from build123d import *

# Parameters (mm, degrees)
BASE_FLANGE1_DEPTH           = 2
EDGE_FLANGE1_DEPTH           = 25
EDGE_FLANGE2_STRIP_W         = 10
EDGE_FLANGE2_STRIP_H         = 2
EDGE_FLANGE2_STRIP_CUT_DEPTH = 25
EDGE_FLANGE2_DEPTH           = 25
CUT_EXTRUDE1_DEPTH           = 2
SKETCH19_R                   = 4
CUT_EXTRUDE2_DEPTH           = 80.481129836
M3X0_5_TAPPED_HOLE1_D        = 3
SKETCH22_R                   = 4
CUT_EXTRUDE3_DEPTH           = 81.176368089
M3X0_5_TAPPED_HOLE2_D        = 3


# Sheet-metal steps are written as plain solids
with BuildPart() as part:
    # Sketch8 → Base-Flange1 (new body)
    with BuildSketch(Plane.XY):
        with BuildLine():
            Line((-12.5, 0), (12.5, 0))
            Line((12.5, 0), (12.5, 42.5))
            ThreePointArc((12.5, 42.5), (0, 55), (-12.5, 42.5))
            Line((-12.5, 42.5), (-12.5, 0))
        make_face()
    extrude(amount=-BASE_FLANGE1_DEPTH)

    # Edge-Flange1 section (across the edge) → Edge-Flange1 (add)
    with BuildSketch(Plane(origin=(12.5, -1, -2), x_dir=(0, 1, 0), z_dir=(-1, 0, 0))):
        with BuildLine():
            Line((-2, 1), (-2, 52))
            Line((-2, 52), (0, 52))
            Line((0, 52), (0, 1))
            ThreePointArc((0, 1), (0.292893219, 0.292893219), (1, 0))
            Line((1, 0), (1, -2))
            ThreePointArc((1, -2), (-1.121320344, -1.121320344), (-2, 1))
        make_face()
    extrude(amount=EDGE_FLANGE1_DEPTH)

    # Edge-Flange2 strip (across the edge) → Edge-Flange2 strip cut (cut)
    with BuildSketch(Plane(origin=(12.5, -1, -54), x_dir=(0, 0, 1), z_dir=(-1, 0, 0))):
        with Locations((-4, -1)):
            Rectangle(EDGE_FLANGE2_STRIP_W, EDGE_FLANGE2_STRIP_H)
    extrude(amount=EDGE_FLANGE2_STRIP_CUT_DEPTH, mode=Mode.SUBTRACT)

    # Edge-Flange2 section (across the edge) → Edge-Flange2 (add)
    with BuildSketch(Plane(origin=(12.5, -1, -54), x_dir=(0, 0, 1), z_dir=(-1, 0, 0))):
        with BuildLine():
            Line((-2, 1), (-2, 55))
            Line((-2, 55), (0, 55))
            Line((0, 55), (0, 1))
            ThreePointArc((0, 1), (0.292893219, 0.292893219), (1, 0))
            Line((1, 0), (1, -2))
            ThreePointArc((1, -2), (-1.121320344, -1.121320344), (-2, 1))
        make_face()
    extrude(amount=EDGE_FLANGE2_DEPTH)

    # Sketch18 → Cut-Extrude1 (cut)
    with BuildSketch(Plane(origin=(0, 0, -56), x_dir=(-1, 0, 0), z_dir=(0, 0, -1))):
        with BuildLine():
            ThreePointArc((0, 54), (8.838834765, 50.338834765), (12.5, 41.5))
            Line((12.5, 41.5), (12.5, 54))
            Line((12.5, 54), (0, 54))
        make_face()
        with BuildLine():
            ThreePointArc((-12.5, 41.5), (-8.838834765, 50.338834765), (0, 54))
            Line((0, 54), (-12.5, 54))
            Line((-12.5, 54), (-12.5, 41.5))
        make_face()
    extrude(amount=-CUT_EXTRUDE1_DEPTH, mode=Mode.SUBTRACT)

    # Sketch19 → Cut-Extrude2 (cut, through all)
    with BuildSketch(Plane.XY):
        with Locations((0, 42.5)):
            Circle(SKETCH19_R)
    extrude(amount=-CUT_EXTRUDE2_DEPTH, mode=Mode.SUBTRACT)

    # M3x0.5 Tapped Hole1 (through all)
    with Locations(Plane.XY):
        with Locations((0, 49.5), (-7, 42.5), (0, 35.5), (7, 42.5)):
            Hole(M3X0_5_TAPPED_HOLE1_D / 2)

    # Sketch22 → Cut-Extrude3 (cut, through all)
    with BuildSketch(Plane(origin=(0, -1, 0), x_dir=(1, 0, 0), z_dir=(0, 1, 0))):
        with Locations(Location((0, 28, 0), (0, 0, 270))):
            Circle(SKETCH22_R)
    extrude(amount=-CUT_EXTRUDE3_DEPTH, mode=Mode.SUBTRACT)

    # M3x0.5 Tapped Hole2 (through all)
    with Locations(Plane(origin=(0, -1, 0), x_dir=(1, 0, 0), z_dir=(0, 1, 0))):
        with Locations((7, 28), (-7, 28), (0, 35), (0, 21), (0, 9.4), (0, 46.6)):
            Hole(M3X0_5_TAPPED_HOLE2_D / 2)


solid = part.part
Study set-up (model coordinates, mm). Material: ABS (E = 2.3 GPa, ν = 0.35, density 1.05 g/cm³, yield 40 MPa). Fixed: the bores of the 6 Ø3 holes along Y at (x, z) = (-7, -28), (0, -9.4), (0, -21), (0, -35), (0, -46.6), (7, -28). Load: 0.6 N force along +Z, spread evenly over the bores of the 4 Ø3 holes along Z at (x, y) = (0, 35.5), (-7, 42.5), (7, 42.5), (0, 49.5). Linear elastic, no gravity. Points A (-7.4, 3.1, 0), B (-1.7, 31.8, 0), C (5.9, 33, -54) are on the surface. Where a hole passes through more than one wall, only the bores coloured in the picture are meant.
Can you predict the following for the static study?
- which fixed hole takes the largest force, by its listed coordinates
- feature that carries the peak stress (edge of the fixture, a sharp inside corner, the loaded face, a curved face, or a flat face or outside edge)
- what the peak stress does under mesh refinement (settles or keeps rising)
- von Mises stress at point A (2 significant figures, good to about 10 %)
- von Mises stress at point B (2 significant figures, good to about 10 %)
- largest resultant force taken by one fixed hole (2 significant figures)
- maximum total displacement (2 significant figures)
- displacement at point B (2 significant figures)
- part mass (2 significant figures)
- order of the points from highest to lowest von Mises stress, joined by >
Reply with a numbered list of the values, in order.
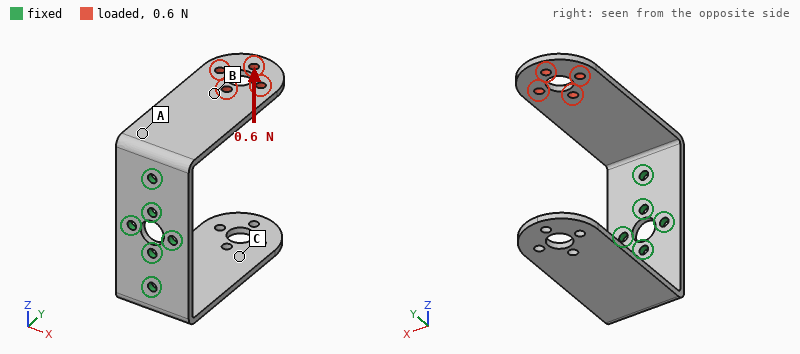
1. (0, -9.4)
2. edge of the fixture
3. keeps rising
4. 1.3 MPa
5. 0.40 MPa
6. 1.1 N
7. 0.93 mm
8. 0.46 mm
9. 7.9 g
10. A > B > C
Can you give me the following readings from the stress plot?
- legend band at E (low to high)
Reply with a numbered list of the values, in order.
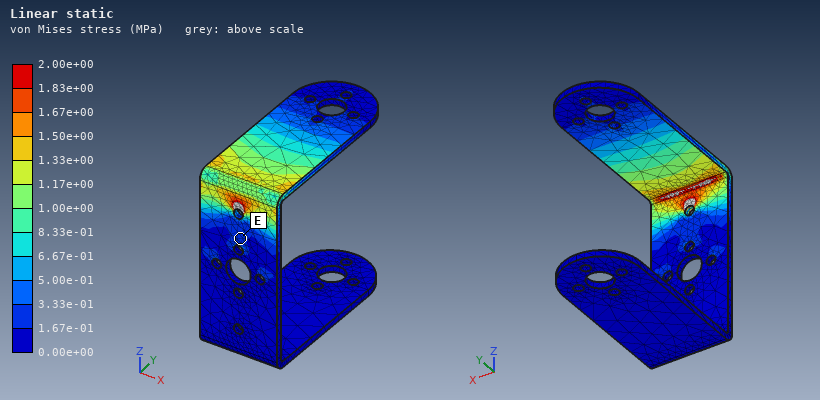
1. 1.67e-01 to 3.33e-01 MPa
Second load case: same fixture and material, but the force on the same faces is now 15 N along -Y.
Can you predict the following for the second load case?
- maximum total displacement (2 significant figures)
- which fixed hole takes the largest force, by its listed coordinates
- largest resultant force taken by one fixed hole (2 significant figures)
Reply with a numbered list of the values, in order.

1. 0.85 mm
2. (0, -9.4)
3. 18 N
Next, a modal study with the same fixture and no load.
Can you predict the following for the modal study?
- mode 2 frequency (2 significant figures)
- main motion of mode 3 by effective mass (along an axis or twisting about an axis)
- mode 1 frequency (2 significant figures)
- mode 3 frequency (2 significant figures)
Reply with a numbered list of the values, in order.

1. 150 Hz
2. along X
3. 140 Hz
4. 270 Hz
